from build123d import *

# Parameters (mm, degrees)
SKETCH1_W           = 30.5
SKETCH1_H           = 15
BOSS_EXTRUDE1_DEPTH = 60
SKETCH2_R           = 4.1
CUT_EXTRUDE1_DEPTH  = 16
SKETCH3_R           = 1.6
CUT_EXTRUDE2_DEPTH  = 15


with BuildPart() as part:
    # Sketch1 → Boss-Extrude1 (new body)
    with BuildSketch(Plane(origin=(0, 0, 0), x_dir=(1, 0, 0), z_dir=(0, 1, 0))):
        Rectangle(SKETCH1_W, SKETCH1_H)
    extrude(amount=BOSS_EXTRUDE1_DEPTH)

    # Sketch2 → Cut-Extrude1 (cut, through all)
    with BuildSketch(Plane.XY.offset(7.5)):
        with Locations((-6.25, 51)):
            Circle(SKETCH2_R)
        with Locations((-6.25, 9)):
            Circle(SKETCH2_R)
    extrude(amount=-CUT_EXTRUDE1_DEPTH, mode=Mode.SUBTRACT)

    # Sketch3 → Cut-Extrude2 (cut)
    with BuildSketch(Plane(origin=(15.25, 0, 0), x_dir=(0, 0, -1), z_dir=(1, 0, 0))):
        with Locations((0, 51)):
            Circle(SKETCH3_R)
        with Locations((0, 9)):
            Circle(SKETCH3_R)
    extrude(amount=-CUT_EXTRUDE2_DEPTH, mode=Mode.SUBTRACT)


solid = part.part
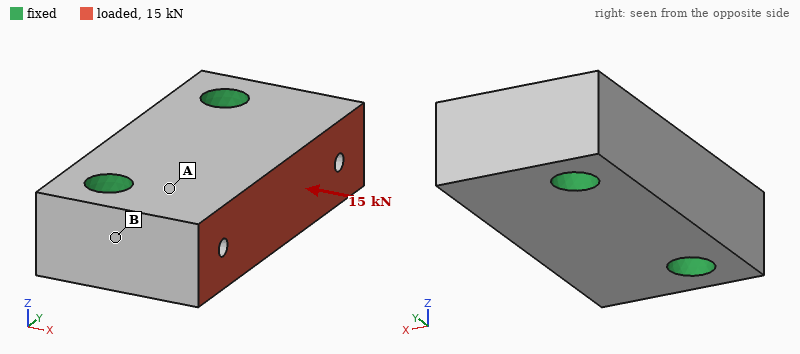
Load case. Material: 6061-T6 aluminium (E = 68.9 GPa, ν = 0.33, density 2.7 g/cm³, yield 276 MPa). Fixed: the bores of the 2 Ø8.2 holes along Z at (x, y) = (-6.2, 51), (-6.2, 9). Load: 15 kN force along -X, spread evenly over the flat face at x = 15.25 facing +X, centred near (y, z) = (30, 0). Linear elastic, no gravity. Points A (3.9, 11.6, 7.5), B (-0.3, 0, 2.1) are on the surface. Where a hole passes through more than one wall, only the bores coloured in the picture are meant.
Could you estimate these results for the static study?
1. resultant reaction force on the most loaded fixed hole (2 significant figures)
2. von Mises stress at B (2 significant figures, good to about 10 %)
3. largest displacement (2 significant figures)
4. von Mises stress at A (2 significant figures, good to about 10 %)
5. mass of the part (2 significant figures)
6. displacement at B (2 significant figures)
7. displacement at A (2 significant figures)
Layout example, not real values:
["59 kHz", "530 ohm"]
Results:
["7.7 kN", "10 MPa", "9.1 µm", "26 MPa", "69 g", "2.1 µm", "3.1 µm"]
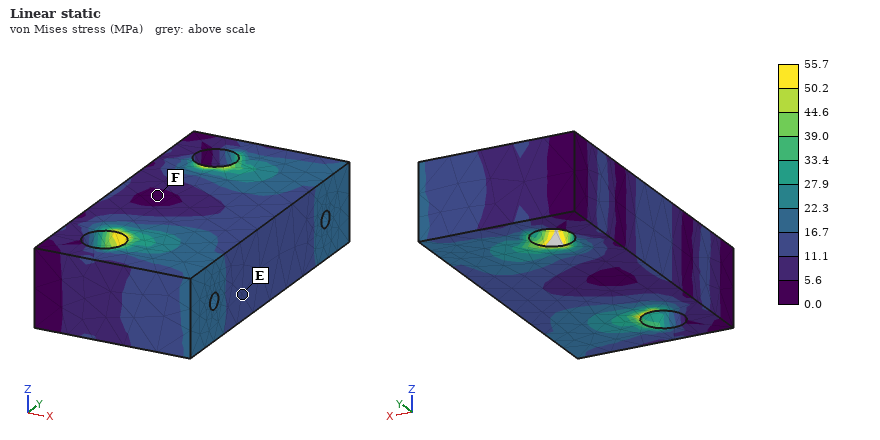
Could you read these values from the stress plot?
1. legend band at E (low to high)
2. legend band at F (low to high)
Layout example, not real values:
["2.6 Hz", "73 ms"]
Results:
["11.1 to 16.7 MPa", "0.0 to 5.6 MPa"]
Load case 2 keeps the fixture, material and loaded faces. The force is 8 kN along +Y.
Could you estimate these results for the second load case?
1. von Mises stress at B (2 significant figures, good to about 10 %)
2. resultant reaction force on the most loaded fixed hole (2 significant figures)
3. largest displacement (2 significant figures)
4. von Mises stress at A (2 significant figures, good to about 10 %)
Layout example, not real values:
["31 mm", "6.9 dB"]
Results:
["20 MPa", "5.2 kN", "15 µm", "19 MPa"]
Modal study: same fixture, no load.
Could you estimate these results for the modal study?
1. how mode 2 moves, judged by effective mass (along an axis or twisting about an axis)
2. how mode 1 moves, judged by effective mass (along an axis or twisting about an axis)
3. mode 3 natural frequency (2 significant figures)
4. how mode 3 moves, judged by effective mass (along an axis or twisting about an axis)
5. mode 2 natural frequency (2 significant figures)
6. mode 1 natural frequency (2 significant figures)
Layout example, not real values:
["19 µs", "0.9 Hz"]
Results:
["twisting about X", "along Z", "30 kHz", "along X", "26 kHz", "18 kHz"]
